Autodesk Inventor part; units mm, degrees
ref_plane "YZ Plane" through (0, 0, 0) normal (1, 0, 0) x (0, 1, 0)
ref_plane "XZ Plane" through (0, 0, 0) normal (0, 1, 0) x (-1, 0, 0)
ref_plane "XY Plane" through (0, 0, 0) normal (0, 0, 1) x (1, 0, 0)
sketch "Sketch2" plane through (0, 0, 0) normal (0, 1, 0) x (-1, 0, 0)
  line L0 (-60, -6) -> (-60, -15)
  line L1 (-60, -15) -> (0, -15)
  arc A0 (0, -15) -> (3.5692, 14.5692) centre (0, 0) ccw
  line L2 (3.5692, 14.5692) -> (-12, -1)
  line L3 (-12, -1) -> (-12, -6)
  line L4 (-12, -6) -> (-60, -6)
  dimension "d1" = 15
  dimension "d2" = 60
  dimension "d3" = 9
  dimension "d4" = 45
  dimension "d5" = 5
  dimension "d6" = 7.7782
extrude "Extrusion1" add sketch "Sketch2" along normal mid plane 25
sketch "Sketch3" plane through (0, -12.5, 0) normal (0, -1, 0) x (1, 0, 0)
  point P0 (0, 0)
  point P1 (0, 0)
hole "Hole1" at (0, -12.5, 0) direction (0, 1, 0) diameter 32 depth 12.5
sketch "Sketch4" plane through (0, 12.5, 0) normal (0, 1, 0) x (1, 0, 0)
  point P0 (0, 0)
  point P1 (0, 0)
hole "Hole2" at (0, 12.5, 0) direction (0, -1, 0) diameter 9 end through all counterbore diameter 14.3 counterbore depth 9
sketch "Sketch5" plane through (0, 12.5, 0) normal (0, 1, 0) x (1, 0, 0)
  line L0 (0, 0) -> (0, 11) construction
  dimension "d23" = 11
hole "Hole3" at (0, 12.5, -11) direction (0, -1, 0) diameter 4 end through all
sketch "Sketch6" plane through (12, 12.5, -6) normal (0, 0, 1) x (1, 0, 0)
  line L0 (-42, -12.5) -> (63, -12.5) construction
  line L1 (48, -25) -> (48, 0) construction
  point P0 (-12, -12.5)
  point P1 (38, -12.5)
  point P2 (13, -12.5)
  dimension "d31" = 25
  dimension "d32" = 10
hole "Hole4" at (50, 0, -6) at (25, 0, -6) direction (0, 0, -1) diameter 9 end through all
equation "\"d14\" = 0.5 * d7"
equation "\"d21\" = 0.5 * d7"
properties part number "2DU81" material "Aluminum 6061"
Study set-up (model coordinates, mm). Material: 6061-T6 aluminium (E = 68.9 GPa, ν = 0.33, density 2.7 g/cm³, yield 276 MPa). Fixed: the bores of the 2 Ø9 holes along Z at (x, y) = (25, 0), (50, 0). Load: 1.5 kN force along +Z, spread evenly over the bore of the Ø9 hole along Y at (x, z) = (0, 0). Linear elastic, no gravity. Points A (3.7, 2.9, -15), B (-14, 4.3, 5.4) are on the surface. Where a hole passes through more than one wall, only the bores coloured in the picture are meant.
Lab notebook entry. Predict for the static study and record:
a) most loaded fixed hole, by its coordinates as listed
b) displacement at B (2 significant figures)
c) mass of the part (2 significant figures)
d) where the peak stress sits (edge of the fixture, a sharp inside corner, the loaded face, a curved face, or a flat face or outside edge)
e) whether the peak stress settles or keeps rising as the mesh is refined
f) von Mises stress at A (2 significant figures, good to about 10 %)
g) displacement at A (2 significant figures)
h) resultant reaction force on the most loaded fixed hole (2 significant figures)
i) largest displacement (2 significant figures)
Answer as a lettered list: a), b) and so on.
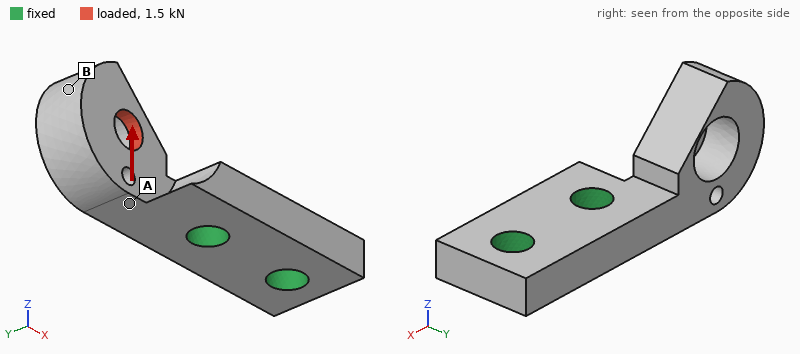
a) (25, 0)
b) 0.20 mm
c) 41 g
d) edge of the fixture
e) keeps rising
f) 39 MPa
g) 0.077 mm
h) 1.7 kN
i) 0.21 mm
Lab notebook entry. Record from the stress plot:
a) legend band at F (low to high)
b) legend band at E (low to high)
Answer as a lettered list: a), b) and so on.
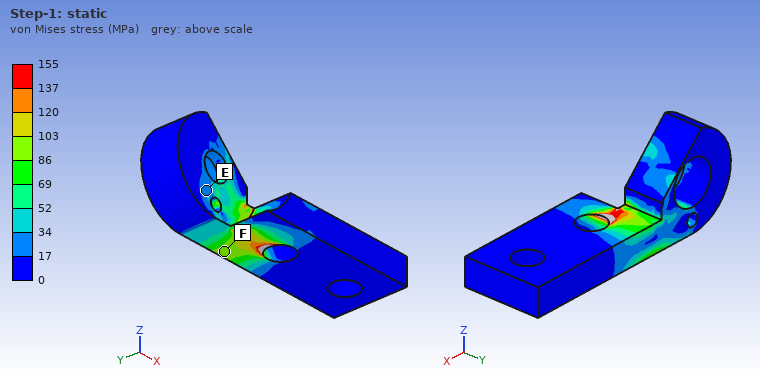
a) 86 to 103 MPa
b) 17 to 34 MPa
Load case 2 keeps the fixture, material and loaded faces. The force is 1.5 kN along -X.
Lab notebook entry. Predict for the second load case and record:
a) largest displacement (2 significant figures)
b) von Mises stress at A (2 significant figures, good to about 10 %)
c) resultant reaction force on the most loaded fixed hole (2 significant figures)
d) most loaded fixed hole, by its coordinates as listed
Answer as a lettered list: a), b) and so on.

a) 0.15 mm
b) 20 MPa
c) 1.4 kN
d) (25, 0)
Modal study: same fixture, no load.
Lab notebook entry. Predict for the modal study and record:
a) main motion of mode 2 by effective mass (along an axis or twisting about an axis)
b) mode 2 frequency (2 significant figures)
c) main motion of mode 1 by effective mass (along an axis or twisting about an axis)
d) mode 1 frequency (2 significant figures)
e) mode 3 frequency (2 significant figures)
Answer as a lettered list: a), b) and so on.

a) along Y
b) 4500 Hz
c) along Z
d) 3500 Hz
e) 11 kHz
